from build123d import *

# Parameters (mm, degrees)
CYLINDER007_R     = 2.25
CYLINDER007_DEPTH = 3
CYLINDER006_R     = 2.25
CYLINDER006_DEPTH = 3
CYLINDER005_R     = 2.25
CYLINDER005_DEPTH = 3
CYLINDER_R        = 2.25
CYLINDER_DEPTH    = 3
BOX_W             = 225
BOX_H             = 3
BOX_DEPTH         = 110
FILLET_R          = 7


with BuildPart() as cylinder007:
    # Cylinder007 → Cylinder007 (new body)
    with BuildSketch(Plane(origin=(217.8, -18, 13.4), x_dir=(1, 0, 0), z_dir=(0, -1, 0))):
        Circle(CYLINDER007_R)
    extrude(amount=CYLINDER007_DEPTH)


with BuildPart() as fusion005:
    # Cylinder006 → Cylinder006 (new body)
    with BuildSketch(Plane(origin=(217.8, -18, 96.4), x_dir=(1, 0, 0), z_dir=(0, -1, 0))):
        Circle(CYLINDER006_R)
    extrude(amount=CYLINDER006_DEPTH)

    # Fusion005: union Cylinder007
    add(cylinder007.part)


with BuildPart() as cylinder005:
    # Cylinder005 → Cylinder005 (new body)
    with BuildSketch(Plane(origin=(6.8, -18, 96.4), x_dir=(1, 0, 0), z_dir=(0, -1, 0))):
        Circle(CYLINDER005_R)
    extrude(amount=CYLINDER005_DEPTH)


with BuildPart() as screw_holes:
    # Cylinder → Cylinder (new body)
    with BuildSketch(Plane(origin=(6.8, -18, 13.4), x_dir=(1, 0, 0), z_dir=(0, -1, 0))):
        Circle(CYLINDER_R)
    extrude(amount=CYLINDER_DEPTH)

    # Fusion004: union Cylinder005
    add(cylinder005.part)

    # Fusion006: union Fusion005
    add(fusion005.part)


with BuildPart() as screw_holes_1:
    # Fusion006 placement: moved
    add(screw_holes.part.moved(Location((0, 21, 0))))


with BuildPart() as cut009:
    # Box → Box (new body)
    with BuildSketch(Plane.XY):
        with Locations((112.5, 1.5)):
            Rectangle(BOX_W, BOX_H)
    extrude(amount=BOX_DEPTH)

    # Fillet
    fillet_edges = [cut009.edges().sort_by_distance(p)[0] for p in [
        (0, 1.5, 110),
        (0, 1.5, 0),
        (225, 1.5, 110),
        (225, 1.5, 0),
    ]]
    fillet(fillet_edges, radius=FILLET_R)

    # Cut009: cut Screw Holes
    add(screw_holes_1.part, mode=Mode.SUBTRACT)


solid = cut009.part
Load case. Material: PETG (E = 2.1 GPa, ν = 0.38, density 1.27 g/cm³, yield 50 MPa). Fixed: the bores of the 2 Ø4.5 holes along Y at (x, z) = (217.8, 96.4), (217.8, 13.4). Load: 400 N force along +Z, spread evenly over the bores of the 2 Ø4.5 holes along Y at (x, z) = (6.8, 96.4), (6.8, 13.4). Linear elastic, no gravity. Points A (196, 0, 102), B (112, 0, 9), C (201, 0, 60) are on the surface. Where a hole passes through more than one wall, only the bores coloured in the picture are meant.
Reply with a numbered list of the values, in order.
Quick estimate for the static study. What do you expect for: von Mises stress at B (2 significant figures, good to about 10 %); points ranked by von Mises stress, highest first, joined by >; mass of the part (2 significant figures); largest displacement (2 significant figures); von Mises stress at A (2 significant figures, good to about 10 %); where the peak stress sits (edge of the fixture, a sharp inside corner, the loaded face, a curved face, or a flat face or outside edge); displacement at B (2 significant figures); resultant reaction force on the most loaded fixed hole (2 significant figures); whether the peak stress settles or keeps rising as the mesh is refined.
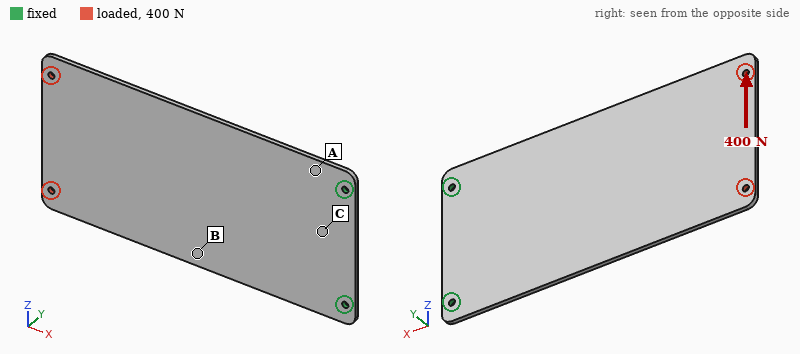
1. 5.9 MPa
2. A > B > C
3. 94 g
4. 2.8 mm
5. 11 MPa
6. edge of the fixture
7. 1.1 mm
8. 1.0 kN
9. keeps rising
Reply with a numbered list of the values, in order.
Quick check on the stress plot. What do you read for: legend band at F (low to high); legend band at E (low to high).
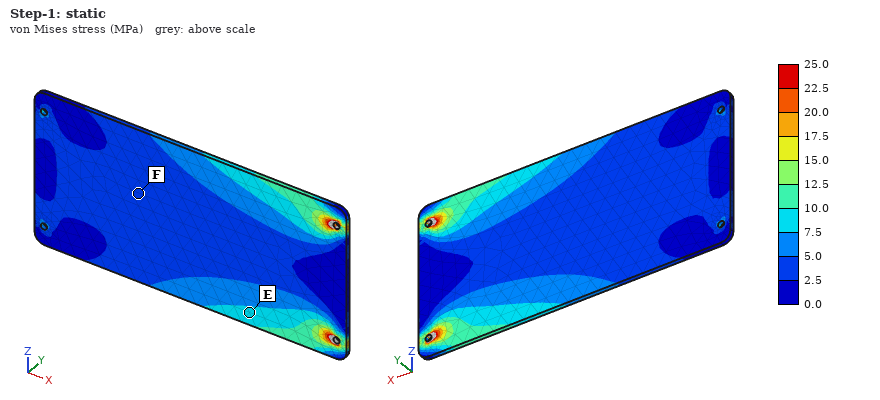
1. 2.5 to 5.0 MPa
2. 7.5 to 10.0 MPa
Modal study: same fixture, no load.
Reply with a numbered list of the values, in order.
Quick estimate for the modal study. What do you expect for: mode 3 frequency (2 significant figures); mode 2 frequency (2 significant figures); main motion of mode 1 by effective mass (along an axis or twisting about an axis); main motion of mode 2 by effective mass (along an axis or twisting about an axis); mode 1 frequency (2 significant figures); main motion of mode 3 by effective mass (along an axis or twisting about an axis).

1. 79 Hz
2. 56 Hz
3. along Y
4. twisting about X
5. 12 Hz
6. along Y
